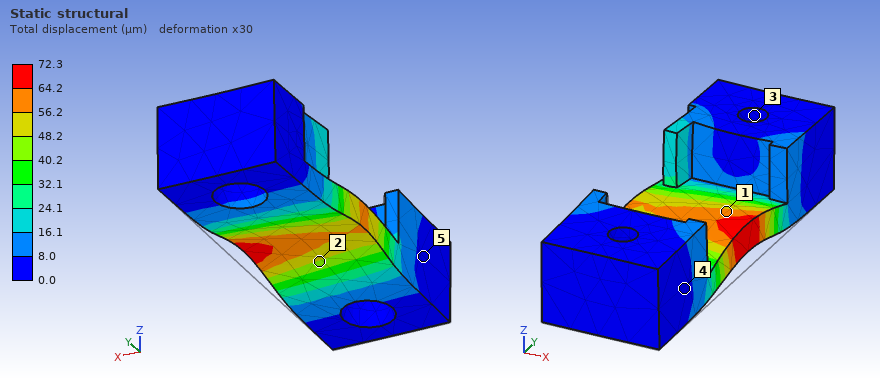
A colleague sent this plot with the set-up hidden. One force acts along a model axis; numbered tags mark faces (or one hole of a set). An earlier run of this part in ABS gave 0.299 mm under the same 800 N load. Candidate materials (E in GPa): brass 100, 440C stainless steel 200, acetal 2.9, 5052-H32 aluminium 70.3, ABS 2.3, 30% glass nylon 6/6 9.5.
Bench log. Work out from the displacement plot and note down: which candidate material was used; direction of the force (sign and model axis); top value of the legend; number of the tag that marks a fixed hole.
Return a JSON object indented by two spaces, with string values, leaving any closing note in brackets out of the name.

{
  "which candidate material was used": "30% glass nylon 6/6",
  "direction of the force": "+Z",
  "top value of the legend": "72.3 µm",
  "number of the tag that marks a fixed hole": "3"
}
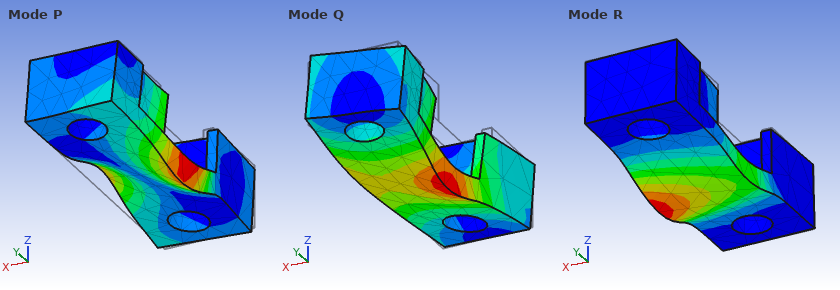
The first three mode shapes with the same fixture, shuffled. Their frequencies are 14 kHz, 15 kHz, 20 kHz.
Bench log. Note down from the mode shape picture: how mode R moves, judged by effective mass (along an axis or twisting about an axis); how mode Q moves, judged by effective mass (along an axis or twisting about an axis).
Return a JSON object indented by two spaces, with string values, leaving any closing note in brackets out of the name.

{
  "how mode R moves, judged by effective mass": "along Z",
  "how mode Q moves, judged by effective mass": "along X"
}
